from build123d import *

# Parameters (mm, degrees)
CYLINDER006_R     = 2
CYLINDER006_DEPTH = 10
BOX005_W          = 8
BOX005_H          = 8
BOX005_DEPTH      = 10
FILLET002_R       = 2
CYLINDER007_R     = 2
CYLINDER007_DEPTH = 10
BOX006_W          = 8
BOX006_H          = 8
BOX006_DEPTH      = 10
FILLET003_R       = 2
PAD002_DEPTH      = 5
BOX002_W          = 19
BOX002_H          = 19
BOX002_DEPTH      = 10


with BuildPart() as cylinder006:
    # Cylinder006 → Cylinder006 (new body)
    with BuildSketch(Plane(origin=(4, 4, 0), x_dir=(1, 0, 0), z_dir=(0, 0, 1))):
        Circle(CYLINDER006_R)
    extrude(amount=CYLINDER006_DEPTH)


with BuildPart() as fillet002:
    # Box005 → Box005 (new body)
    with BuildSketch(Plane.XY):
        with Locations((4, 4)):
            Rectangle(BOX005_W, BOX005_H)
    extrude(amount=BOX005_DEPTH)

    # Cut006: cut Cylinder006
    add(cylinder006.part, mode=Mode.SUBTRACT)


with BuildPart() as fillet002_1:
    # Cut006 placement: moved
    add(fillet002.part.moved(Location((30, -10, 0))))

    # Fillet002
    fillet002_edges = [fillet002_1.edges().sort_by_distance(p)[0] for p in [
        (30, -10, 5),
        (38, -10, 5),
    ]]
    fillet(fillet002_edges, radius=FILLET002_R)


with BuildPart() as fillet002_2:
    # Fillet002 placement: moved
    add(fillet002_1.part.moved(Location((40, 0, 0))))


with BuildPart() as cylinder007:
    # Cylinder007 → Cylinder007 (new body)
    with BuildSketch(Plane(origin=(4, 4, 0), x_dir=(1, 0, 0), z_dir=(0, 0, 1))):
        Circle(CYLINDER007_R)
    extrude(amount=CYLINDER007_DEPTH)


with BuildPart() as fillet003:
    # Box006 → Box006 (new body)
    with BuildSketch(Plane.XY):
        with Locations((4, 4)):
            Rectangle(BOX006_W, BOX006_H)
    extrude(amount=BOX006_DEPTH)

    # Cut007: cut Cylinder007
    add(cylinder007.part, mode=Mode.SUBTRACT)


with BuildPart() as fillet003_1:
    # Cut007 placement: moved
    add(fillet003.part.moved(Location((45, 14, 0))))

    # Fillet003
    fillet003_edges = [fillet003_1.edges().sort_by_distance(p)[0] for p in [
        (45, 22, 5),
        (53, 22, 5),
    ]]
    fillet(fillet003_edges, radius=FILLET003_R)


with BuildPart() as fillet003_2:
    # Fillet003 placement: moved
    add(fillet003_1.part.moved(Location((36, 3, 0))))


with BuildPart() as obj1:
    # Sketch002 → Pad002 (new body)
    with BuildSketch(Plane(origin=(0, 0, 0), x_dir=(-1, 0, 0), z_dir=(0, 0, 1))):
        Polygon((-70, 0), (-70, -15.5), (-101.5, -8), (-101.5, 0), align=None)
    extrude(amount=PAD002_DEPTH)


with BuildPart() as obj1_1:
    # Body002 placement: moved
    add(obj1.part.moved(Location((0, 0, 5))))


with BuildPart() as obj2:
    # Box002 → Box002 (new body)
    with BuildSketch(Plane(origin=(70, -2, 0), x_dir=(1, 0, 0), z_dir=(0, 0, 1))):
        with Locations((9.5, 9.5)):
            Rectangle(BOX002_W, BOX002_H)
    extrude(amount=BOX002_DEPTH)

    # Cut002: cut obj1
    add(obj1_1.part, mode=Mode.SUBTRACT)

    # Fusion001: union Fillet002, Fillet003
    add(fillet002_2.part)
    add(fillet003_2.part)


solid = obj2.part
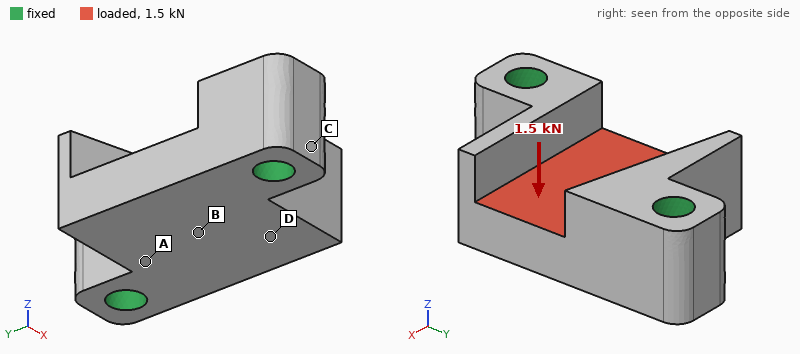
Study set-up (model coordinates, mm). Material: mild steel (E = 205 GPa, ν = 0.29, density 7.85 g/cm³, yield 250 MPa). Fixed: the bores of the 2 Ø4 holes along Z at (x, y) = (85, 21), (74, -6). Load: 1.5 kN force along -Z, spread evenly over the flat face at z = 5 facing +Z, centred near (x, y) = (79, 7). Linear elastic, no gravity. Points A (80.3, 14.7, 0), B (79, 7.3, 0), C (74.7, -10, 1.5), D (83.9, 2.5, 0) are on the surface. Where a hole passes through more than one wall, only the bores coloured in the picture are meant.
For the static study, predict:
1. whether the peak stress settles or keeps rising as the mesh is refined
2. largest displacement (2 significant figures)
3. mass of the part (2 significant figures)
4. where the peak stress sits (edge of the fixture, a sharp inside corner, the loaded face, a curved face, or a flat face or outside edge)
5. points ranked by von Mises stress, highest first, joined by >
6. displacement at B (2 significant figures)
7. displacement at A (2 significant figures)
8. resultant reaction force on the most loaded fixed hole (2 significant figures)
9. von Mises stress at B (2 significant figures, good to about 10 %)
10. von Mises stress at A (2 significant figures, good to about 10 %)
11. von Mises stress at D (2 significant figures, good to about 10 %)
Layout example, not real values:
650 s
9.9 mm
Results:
keeps rising
4.5 µm
26 g
edge of the fixture
B > D > A > C
3.0 µm
1.9 µm
820 N
34 MPa
13 MPa
24 MPa
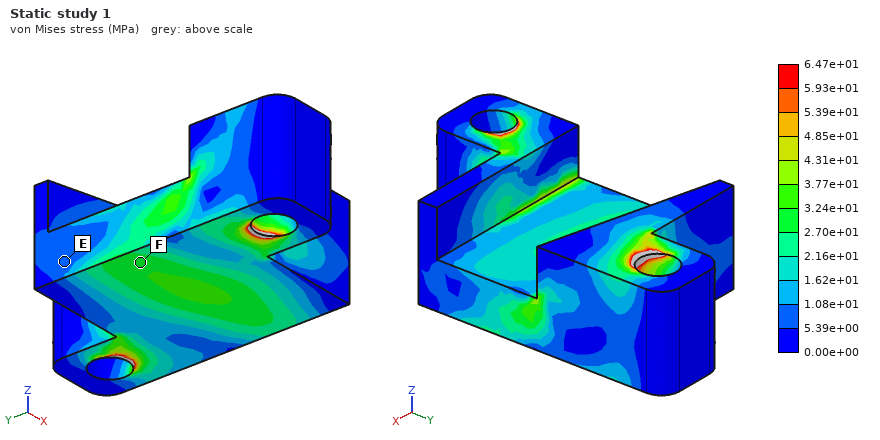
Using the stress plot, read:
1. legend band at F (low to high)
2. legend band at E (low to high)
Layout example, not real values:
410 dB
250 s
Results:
2.70e+01 to 3.24e+01 MPa
5.39e+00 to 1.08e+01 MPa
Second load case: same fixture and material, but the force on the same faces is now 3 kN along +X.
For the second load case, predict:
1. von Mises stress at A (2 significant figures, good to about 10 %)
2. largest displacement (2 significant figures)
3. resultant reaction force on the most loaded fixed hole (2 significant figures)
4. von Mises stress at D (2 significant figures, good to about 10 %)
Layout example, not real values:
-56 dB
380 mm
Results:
22 MPa
5.2 µm
1.6 kN
18 MPa
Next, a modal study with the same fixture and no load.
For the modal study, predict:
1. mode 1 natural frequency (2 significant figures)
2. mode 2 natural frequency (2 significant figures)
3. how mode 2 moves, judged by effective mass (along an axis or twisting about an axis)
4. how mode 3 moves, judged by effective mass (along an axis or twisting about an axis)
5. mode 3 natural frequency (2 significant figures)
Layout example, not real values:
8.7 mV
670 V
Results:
25 kHz
29 kHz
along Z
along X
38 kHz
